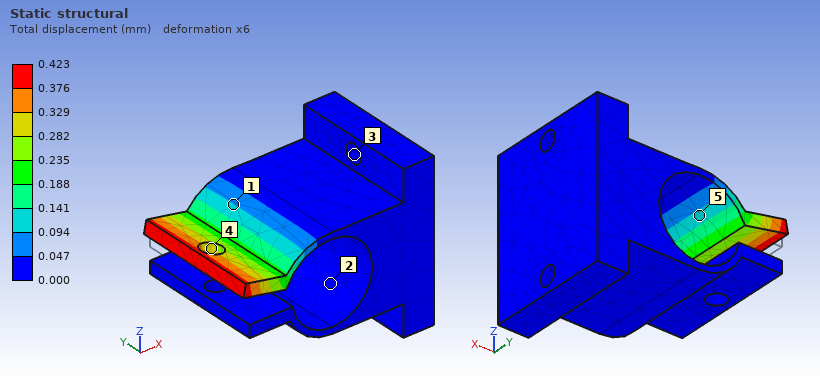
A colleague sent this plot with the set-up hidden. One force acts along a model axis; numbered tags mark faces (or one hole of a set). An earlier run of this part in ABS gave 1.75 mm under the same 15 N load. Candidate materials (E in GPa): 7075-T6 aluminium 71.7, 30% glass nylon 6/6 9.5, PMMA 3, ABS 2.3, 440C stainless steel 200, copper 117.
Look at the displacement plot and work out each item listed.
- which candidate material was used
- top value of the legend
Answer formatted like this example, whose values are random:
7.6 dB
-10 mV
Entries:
30% glass nylon 6/6
0.423 mm
